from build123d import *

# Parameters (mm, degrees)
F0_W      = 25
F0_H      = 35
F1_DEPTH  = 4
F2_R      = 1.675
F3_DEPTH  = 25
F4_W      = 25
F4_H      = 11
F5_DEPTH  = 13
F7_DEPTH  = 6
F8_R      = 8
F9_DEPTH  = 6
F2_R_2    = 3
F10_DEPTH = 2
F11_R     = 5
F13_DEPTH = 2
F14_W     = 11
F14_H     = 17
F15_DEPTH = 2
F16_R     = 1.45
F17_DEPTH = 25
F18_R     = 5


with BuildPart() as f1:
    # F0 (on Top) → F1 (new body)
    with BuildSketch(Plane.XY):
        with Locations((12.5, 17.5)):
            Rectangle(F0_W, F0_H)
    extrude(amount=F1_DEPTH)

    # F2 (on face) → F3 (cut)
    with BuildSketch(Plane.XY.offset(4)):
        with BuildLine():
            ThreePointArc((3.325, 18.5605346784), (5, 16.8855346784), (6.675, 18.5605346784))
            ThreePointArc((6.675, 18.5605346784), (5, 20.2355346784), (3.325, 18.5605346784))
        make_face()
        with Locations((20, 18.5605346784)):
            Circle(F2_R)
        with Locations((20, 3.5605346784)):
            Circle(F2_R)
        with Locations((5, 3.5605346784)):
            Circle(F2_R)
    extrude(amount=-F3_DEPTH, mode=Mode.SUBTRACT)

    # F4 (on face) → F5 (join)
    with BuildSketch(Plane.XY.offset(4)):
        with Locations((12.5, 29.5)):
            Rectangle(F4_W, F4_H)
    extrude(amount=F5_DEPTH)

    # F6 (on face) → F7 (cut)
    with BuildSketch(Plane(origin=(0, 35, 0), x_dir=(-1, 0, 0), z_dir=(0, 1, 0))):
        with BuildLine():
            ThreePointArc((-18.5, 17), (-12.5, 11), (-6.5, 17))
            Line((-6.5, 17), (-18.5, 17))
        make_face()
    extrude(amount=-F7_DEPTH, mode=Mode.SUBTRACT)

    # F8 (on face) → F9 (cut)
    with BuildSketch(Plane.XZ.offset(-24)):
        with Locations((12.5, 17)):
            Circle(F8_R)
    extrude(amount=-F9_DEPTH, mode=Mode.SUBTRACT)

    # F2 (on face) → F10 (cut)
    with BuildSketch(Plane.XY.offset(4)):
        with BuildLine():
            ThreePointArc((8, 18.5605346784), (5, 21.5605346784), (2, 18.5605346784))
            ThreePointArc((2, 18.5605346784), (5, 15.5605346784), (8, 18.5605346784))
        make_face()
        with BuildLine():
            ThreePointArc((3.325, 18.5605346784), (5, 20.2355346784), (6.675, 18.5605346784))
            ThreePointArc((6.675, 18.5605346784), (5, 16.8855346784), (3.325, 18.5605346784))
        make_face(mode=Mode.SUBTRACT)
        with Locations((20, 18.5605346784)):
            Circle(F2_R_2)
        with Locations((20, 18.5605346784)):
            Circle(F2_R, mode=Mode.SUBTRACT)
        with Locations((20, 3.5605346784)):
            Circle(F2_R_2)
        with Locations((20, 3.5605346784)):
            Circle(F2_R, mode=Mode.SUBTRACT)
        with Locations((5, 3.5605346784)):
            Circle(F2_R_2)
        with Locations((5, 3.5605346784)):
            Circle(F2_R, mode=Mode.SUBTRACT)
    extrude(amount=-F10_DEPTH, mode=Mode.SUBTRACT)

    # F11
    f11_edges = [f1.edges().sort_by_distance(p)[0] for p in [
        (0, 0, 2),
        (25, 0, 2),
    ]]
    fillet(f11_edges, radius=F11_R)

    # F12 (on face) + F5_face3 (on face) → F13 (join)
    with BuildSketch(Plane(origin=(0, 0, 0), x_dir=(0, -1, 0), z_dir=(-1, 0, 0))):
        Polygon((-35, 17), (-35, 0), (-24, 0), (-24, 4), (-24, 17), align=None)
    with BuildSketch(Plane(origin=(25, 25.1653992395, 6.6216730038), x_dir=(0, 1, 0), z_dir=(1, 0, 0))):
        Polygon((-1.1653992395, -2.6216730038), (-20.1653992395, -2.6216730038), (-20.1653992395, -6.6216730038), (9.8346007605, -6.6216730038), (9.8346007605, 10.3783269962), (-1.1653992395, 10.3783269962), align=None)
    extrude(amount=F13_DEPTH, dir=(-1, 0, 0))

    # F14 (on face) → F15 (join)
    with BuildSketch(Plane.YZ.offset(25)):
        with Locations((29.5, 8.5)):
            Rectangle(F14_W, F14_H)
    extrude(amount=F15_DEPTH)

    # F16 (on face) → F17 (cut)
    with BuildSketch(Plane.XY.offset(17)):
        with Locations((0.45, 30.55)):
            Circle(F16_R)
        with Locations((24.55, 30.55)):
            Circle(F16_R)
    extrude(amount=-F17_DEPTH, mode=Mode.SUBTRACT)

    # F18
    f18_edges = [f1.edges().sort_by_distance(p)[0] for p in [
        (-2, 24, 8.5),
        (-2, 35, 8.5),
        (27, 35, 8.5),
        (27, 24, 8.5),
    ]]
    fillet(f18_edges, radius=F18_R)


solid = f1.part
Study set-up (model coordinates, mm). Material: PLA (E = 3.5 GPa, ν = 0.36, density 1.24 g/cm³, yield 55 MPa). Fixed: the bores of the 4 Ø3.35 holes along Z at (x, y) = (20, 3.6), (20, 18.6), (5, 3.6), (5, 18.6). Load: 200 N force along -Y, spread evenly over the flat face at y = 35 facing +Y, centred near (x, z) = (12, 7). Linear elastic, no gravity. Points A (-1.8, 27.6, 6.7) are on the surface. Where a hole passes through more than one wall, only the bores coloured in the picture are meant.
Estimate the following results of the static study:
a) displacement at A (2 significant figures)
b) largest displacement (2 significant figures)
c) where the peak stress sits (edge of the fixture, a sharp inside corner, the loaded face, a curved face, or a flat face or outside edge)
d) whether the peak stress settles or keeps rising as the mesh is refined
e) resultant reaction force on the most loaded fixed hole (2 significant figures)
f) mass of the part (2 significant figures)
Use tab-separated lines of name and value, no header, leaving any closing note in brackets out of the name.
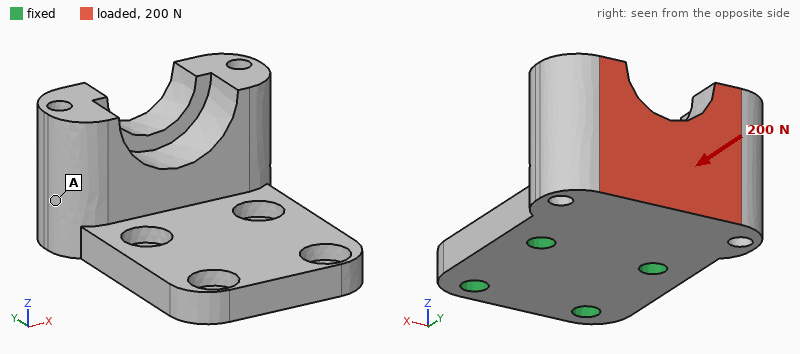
displacement at A	0.20 mm
largest displacement	0.52 mm
where the peak stress sits	edge of the fixture
whether the peak stress settles or keeps rising as the mesh is refined	keeps rising
resultant reaction force on the most loaded fixed hole	72 N
mass of the part	7.5 g
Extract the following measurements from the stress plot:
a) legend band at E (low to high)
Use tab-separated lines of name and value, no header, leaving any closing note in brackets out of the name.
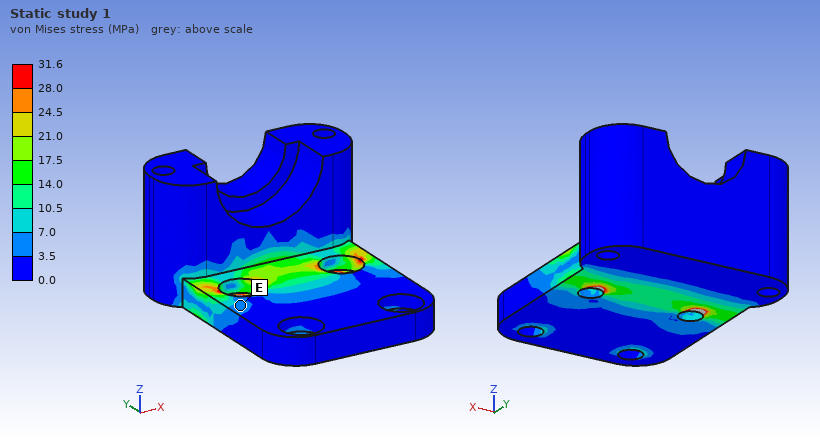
legend band at E	3.5 to 7.0 MPa
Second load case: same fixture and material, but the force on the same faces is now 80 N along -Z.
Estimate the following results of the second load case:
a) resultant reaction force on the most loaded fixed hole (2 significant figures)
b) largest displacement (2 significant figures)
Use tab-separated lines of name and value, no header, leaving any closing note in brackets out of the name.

resultant reaction force on the most loaded fixed hole	82 N
largest displacement	0.50 mm
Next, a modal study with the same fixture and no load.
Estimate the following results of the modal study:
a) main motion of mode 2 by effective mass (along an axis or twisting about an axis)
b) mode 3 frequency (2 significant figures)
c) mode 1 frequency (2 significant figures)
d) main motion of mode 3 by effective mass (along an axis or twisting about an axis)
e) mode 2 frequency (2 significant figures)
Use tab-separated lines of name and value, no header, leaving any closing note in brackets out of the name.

main motion of mode 2 by effective mass	along X
mode 3 frequency	5500 Hz
mode 1 frequency	1300 Hz
main motion of mode 3 by effective mass	along X
mode 2 frequency	3300 Hz
